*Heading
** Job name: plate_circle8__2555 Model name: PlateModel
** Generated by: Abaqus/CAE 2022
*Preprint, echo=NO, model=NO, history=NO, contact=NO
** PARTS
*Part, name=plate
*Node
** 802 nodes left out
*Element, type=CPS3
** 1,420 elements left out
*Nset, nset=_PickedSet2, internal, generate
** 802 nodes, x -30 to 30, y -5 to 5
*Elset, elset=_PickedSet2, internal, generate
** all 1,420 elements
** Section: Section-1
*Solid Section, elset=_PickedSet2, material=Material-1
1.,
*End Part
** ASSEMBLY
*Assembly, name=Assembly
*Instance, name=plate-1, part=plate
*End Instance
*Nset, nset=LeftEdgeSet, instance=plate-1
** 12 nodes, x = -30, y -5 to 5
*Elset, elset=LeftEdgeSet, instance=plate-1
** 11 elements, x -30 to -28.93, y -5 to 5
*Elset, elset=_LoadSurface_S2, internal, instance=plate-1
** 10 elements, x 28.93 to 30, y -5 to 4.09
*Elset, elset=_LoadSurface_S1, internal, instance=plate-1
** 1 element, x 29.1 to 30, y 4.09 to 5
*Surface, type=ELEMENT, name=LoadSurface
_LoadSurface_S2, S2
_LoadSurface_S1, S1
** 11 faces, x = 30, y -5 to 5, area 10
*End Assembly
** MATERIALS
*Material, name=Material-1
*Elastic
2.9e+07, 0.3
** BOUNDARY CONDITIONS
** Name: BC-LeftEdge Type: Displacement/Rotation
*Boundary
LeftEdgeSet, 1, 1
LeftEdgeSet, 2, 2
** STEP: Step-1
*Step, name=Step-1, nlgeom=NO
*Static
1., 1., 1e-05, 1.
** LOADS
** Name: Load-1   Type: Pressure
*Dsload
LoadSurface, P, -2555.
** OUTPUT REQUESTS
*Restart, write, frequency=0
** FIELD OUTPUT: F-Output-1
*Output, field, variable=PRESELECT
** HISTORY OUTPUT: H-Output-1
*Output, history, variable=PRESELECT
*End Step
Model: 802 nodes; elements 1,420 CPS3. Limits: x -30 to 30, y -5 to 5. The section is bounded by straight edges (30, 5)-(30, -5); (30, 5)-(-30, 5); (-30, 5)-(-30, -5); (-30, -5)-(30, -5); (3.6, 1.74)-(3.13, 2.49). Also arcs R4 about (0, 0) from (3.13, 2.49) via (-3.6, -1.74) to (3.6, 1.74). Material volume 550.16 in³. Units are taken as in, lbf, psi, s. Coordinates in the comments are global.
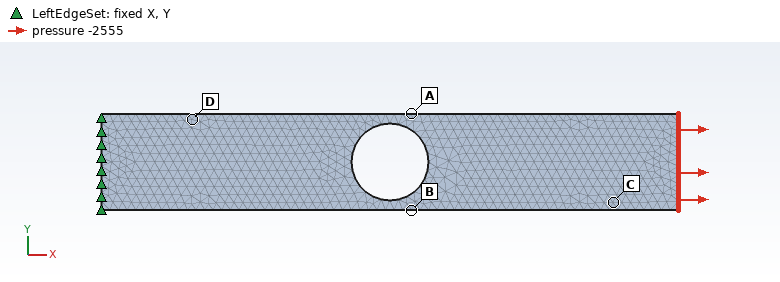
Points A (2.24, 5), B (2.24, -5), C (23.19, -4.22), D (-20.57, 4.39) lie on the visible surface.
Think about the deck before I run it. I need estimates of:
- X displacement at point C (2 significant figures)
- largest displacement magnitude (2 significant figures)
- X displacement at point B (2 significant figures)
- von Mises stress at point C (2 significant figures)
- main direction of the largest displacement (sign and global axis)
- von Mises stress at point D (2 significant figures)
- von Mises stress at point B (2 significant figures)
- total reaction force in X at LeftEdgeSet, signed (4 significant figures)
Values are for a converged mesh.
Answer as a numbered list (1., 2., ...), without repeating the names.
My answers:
1. 0.0080 in
2. 0.0086 in
3. 0.0048 in
4. 2600 psi
5. +X
6. 2500 psi
7. 11000 psi
8. -25550 lbf
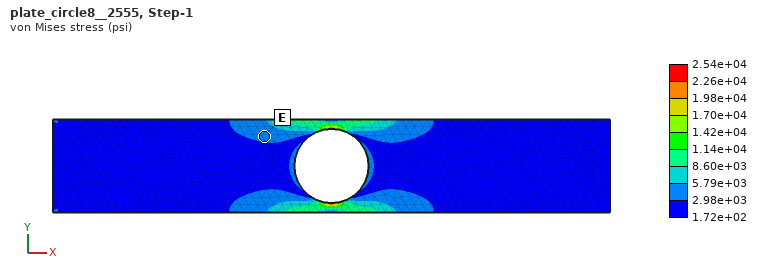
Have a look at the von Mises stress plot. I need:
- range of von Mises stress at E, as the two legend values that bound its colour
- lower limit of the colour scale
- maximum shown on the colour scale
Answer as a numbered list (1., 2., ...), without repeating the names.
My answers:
1. 2.98e+03 to 5.79e+03 psi
2. 1.72e+02 psi
3. 2.54e+04 psi
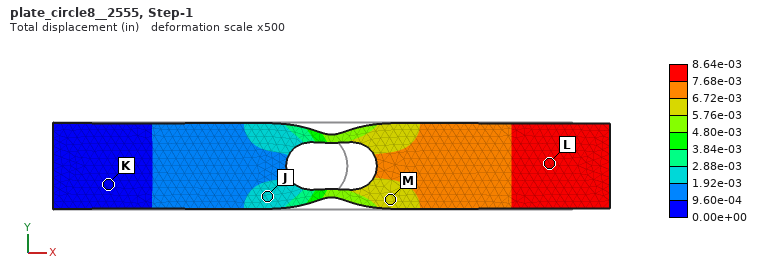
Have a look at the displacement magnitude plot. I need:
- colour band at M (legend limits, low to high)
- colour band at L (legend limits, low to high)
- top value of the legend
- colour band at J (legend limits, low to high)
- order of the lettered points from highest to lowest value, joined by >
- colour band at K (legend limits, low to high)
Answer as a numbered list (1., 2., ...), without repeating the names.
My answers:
1. 5.76e-03 to 6.72e-03 in
2. 7.68e-03 to 8.64e-03 in
3. 8.64e-03 in
4. 1.92e-03 to 2.88e-03 in
5. L > M > J > K
6. 0.00e+00 to 9.60e-04 in
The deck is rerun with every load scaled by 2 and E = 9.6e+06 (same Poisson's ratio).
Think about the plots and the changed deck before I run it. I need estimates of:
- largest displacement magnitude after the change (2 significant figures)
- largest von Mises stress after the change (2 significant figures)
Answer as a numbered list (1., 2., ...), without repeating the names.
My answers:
1. 0.052 in
2. 51000 psi
